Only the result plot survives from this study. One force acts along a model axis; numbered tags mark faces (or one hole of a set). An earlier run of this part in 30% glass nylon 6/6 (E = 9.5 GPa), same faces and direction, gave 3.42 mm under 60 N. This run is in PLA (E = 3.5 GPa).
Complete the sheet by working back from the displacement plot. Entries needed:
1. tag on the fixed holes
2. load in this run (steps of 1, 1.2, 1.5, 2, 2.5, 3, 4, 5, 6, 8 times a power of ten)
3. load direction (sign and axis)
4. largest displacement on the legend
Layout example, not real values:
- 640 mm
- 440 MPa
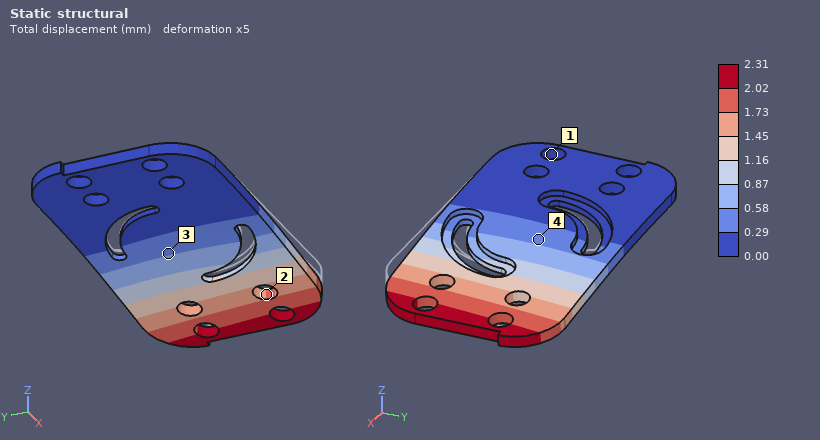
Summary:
- 1
- 15 N
- -Z
- 2.31 mm
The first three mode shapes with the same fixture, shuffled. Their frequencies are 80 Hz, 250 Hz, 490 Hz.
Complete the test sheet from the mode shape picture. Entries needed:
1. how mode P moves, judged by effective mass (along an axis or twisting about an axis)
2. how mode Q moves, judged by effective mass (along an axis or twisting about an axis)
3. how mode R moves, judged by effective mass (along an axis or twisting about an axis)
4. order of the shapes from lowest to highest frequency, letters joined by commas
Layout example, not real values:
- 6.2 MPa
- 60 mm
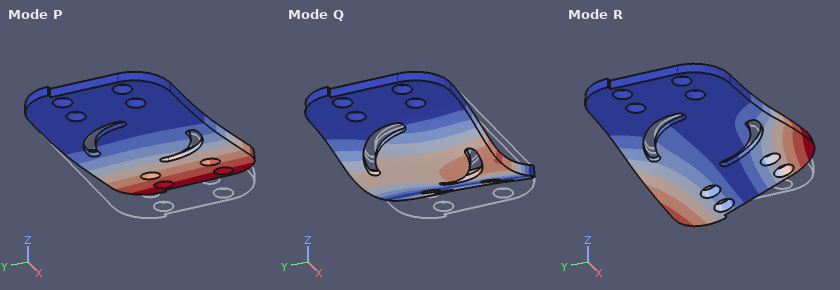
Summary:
- along Z
- along Z
- twisting about X
- P, R, Q
